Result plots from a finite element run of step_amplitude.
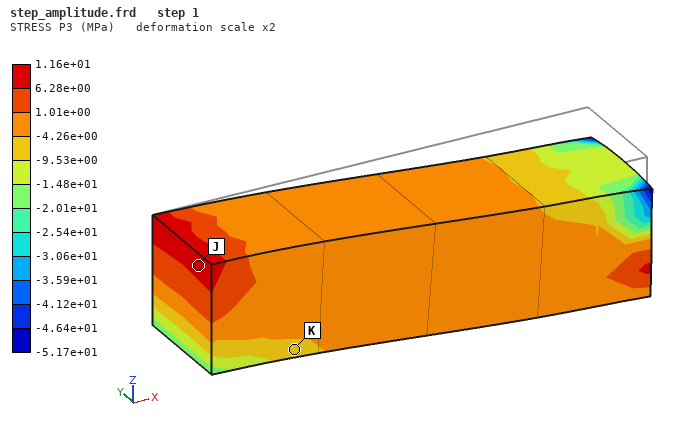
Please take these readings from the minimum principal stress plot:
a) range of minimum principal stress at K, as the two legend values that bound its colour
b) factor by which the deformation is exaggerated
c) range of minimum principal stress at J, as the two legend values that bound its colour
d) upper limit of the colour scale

-9.53e+00 to -4.26e+00 MPa
2
6.28e+00 to 1.16e+01 MPa
1.16e+01 MPa
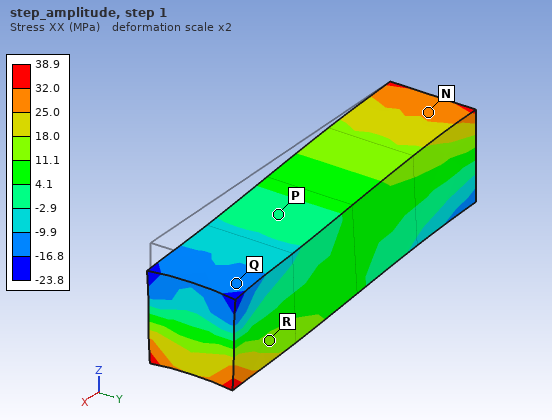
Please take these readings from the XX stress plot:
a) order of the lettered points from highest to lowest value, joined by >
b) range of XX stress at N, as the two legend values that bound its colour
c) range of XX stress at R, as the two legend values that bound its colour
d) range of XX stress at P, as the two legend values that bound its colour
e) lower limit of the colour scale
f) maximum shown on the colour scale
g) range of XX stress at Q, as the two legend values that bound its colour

N > R > P > Q
25.0 to 32.0 MPa
11.1 to 18.0 MPa
-2.9 to 4.1 MPa
-23.8 MPa
38.9 MPa
-16.8 to -9.9 MPa
